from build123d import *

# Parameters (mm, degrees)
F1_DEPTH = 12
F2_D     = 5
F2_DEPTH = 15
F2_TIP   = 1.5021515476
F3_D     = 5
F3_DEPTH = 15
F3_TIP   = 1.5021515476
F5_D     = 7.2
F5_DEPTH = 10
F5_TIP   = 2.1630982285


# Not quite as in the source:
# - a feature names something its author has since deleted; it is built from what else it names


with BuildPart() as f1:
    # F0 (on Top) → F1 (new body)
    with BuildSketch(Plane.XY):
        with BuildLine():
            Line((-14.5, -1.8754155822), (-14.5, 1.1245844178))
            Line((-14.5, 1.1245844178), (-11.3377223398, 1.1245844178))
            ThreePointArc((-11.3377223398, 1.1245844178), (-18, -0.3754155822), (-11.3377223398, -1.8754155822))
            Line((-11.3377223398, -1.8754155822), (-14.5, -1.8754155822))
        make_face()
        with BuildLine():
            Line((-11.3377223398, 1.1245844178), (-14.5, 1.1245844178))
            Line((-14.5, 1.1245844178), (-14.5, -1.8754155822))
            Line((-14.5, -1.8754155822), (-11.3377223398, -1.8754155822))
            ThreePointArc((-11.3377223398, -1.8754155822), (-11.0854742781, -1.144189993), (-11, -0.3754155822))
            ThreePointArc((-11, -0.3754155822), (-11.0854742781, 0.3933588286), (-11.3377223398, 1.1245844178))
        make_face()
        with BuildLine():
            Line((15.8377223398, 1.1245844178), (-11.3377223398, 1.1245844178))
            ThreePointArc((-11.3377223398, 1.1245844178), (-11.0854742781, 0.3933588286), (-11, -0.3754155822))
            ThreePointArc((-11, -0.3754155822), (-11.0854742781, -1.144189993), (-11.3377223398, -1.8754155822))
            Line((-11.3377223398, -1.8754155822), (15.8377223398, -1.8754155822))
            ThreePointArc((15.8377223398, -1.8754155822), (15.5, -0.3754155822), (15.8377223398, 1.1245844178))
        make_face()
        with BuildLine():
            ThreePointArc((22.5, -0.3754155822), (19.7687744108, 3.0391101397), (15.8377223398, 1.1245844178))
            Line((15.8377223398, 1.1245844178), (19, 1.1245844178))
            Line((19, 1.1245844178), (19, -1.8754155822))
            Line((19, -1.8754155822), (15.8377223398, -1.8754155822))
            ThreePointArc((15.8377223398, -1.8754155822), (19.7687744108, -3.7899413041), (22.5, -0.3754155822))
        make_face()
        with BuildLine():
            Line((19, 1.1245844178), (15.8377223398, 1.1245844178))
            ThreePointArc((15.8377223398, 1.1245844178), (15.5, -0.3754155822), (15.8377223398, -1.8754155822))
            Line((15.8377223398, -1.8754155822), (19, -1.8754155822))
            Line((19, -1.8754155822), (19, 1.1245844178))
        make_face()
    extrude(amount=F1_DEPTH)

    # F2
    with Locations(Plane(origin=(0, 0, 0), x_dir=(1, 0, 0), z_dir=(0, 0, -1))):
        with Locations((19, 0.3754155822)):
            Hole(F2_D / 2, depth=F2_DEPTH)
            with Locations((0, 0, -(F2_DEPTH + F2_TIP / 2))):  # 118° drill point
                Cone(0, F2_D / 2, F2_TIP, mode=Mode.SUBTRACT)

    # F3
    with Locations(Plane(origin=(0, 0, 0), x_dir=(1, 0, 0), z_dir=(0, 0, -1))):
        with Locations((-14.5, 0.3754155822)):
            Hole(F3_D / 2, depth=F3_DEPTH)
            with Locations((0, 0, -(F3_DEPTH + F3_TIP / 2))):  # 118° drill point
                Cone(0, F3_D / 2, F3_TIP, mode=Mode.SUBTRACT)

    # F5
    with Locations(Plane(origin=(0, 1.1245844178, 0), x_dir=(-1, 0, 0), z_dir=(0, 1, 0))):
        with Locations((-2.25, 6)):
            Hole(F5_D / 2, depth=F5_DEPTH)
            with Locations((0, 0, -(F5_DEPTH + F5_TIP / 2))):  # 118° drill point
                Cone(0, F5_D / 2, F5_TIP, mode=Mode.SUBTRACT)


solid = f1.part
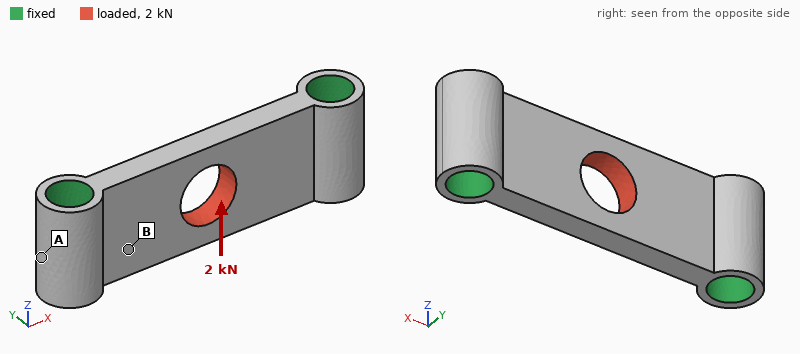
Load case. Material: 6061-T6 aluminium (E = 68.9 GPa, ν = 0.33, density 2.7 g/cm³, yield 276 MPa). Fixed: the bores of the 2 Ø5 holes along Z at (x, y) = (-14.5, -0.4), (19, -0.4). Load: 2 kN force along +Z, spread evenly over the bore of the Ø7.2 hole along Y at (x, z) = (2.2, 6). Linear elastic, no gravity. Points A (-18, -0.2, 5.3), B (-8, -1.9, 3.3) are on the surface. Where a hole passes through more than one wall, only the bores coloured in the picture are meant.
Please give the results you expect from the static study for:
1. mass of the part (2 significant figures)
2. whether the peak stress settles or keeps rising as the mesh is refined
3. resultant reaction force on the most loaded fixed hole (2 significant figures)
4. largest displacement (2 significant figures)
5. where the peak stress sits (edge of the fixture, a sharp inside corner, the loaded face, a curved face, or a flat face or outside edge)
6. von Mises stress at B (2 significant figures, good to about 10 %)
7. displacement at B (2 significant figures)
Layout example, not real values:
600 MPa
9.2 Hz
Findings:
3.5 g
keeps rising
1.0 kN
26 µm
edge of the fixture
61 MPa
6.5 µm
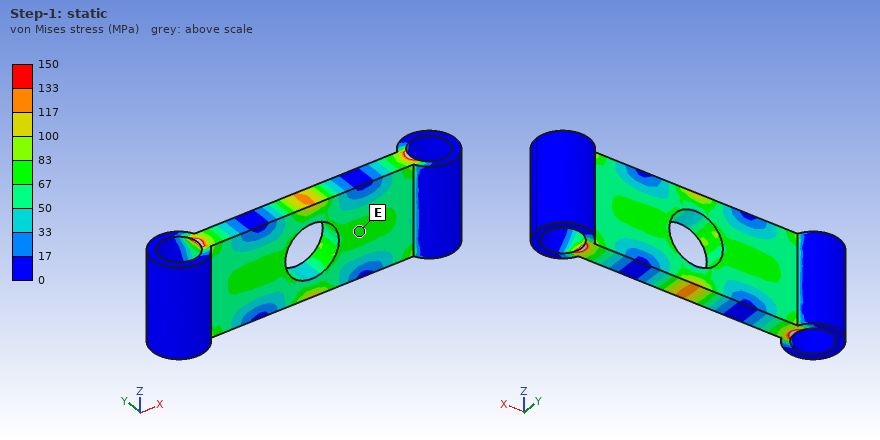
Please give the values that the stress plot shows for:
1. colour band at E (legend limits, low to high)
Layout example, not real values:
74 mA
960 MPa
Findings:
67 to 83 MPa
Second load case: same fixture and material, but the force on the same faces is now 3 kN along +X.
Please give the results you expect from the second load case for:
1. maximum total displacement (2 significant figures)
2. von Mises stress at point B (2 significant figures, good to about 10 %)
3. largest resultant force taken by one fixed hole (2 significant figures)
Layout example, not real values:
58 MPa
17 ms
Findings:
8.7 µm
42 MPa
1.5 kN
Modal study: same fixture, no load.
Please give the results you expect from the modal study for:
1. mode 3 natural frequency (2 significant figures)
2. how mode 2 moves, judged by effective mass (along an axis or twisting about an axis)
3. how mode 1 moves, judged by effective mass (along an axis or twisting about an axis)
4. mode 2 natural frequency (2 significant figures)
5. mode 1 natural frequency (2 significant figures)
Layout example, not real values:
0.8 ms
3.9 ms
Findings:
44 kHz
twisting about X
along Y
30 kHz
19 kHz
